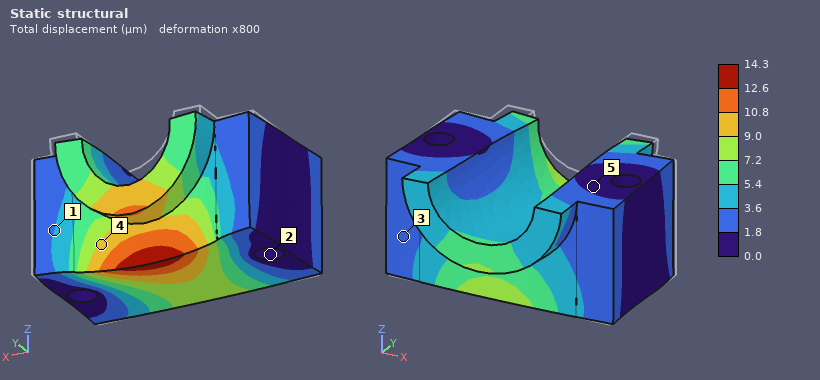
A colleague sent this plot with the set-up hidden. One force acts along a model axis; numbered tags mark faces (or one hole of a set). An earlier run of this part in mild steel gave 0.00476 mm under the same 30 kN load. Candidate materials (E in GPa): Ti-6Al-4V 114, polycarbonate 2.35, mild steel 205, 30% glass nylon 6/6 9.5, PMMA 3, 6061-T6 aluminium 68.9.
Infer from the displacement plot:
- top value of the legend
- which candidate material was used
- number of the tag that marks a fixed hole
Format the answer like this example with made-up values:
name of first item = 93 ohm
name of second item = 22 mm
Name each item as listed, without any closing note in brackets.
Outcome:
top value of the legend = 14.3 µm
which candidate material was used = 6061-T6 aluminium
number of the tag that marks a fixed hole = 2
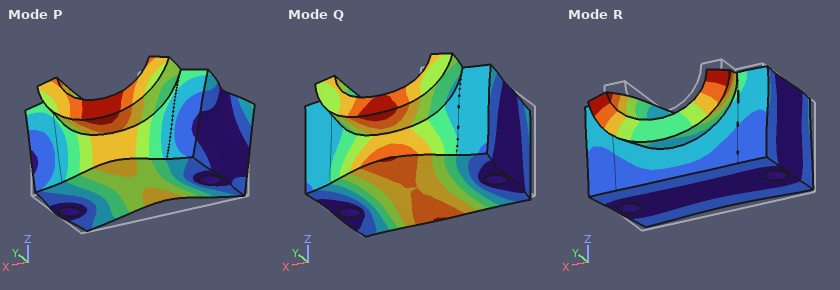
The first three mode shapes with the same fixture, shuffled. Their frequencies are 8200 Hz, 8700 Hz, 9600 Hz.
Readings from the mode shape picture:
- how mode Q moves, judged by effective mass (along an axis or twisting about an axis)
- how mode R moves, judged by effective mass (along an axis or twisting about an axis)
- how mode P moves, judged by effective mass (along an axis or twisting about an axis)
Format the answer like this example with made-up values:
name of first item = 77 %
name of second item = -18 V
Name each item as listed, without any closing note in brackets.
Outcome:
how mode Q moves, judged by effective mass = along Y
how mode R moves, judged by effective mass = along Y
how mode P moves, judged by effective mass = along Z
